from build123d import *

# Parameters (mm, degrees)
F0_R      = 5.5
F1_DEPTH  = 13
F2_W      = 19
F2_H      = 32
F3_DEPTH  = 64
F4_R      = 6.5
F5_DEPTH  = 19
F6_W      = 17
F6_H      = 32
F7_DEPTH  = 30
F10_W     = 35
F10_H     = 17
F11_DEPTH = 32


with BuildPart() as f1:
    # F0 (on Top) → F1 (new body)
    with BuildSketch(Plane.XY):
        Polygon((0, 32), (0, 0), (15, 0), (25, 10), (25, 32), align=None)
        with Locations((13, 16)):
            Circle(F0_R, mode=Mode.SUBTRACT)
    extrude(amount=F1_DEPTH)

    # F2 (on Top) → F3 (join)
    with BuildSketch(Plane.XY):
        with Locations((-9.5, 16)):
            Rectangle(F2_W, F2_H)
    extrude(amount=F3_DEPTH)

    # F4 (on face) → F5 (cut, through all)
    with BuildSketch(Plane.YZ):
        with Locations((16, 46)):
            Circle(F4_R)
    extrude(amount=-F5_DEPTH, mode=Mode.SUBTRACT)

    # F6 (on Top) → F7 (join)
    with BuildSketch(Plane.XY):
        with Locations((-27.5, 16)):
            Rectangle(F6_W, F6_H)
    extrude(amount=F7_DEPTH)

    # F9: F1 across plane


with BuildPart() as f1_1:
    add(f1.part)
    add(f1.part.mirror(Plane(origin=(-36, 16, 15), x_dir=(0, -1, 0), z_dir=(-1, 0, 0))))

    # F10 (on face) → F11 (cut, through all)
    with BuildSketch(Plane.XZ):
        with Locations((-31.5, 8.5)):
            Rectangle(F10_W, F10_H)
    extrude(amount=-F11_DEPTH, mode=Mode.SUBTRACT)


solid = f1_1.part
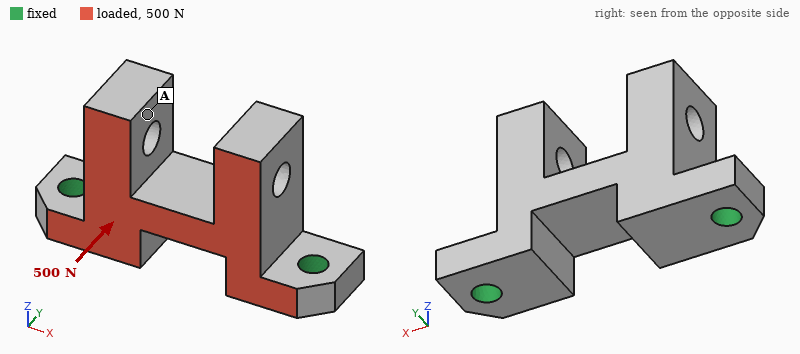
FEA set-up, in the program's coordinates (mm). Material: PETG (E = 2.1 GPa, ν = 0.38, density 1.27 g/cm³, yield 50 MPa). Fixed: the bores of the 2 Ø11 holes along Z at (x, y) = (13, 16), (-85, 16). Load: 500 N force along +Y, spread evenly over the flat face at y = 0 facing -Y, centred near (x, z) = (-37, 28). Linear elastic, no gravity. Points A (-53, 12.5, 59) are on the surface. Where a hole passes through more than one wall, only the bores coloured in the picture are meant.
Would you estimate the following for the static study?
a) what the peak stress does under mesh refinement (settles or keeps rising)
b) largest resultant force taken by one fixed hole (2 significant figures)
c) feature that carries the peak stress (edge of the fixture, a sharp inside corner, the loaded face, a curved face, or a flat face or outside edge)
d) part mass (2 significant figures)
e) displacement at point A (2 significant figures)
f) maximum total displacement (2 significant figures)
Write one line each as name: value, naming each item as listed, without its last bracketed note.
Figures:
what the peak stress does under mesh refinement: keeps rising
largest resultant force taken by one fixed hole: 250 N
feature that carries the peak stress: edge of the fixture
part mass: 130 g
displacement at point A: 0.32 mm
maximum total displacement: 0.37 mm
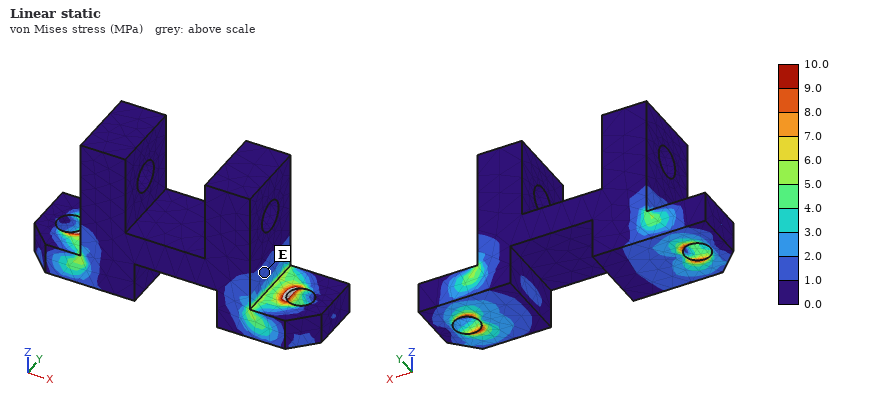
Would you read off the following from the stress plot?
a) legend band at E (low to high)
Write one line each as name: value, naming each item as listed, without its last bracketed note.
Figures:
legend band at E: 1.0 to 2.0 MPa
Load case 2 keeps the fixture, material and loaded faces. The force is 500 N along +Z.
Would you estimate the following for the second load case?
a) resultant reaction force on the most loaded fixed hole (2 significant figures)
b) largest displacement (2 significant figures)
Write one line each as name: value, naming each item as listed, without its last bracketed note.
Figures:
resultant reaction force on the most loaded fixed hole: 300 N
largest displacement: 0.24 mm
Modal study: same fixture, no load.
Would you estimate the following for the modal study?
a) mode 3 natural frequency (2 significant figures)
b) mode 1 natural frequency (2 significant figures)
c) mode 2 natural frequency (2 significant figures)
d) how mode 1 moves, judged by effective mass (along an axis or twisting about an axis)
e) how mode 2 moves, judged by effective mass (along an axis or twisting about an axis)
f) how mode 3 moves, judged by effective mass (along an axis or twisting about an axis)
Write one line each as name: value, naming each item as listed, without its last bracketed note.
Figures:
mode 3 natural frequency: 1300 Hz
mode 1 natural frequency: 670 Hz
mode 2 natural frequency: 1100 Hz
how mode 1 moves, judged by effective mass: along Y
how mode 2 moves, judged by effective mass: twisting about Z
how mode 3 moves, judged by effective mass: along X
